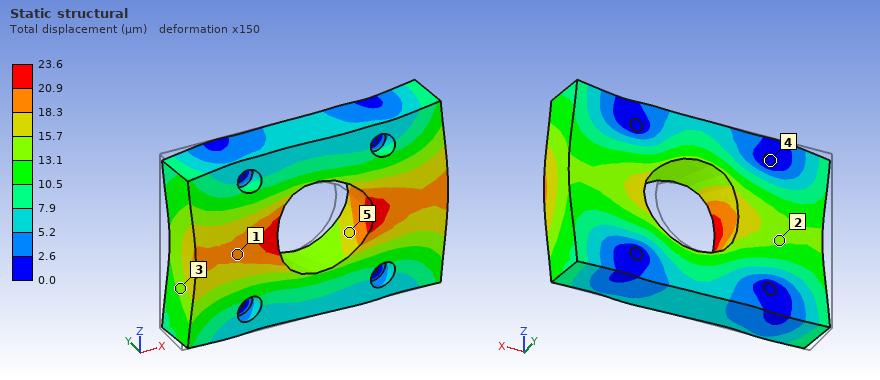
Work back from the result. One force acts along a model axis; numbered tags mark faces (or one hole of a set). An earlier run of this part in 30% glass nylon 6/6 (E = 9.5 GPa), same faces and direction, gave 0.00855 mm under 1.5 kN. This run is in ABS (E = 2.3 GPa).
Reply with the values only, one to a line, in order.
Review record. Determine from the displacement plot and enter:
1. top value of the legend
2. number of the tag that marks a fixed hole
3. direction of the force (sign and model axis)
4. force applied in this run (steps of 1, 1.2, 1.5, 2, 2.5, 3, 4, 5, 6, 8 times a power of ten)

23.6 µm
4
+X
1 kN
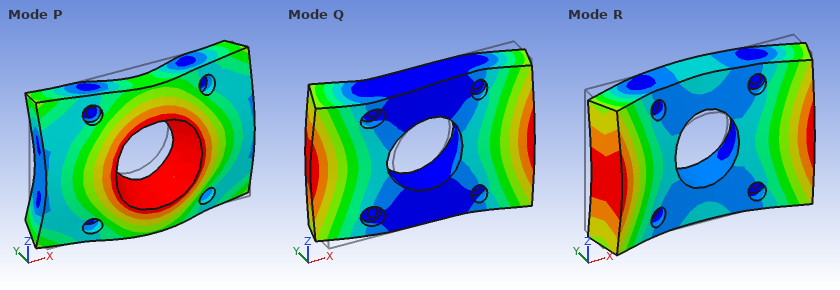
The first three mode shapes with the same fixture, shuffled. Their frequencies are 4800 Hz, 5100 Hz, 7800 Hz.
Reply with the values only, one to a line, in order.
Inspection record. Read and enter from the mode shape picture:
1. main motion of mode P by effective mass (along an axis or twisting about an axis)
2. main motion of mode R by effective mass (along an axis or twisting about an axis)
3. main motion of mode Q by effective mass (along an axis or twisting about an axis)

along Y
along Y
twisting about Z
